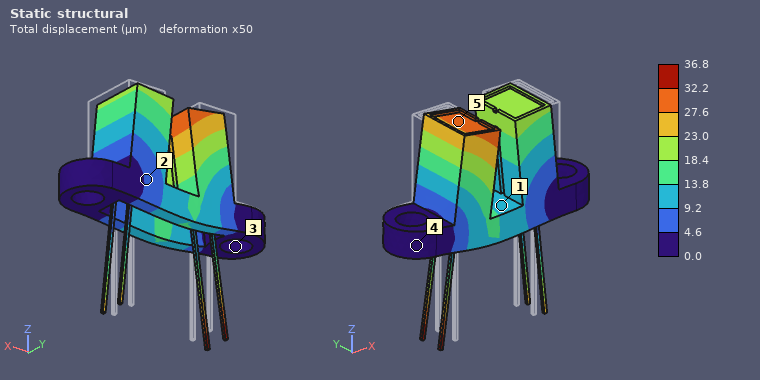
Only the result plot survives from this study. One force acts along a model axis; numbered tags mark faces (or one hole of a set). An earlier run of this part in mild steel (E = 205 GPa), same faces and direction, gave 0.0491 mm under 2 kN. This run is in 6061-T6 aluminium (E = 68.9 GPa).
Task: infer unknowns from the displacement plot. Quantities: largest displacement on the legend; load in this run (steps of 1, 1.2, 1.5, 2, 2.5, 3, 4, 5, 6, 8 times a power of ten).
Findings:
36.8 µm
500 N
